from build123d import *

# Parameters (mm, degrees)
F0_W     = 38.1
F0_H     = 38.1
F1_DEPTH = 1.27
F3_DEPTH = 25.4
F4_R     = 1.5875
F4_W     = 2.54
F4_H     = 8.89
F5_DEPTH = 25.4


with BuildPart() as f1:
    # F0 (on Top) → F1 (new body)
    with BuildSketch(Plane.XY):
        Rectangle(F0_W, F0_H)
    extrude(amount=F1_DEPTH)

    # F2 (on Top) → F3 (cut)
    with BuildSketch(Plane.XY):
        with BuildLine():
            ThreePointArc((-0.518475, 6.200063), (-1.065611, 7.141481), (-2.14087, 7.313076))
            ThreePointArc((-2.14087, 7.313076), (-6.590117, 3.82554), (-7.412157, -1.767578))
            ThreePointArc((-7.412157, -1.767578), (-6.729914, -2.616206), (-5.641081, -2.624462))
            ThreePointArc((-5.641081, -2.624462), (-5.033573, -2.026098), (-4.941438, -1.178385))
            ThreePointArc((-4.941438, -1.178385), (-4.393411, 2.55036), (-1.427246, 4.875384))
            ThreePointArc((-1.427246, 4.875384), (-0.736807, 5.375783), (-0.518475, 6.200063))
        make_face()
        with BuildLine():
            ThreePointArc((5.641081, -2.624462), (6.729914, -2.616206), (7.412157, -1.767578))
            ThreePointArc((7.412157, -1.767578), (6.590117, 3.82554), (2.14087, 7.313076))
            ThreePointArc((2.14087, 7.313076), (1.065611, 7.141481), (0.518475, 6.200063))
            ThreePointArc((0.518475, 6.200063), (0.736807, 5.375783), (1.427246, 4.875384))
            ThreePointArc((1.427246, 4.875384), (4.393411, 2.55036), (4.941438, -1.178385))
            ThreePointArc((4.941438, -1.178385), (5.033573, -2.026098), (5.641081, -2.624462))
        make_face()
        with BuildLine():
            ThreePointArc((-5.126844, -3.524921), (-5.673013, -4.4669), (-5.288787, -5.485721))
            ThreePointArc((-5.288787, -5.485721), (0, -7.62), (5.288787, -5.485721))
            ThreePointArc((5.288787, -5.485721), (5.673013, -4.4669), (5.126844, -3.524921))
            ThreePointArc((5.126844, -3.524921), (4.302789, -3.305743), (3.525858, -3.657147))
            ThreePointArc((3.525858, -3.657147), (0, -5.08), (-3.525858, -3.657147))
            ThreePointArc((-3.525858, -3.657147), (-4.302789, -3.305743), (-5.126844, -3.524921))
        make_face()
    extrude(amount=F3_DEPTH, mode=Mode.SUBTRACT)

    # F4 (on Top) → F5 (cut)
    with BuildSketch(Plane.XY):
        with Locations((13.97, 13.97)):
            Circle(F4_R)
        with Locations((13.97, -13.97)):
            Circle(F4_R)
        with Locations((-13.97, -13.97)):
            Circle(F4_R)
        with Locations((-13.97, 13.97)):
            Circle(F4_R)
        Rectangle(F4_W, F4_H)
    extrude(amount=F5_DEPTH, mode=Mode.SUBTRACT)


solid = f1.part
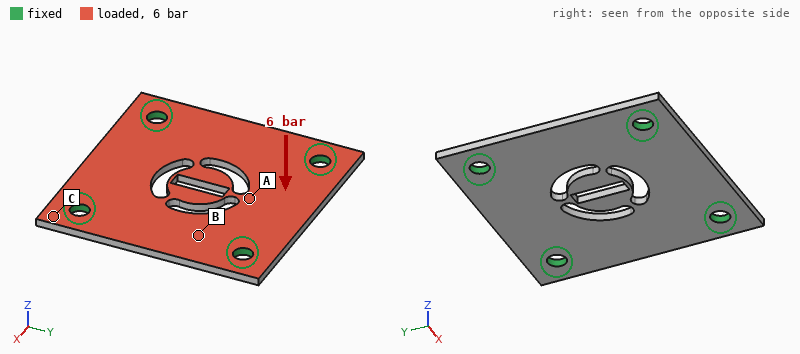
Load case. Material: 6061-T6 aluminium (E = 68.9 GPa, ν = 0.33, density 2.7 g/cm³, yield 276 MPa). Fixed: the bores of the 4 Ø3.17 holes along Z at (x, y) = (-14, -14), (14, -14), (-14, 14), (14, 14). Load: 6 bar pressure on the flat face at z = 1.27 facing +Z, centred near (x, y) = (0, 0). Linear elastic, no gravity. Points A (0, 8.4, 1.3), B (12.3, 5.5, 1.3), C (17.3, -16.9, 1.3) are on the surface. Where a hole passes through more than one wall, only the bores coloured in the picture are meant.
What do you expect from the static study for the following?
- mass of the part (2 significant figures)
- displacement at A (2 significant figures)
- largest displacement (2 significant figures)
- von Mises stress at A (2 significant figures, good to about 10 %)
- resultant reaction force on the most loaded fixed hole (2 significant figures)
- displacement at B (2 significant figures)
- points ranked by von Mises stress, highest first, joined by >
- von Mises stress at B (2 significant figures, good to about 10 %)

4.5 g
0.13 mm
0.18 mm
99 MPa
200 N
0.063 mm
A > B > C
52 MPa
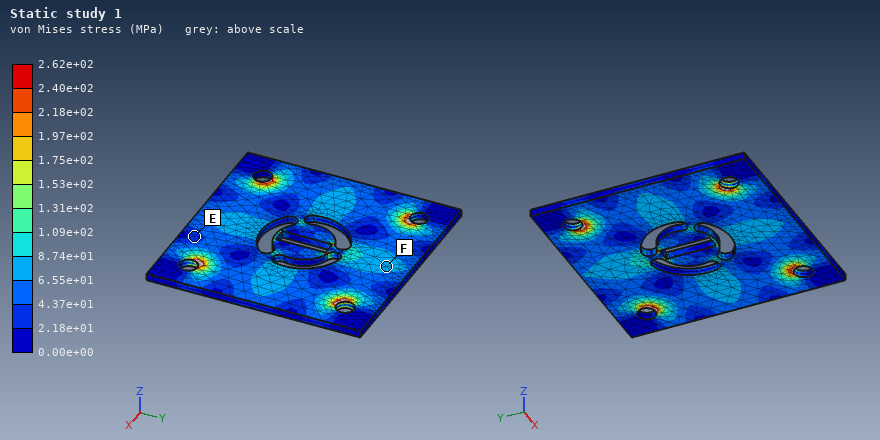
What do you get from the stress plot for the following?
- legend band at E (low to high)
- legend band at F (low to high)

2.18e+01 to 4.37e+01 MPa
6.55e+01 to 8.74e+01 MPa
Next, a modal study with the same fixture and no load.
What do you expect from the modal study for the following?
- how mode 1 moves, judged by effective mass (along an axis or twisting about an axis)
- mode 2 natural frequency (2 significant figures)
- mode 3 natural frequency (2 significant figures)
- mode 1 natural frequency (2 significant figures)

along Z
9900 Hz
9900 Hz
6600 Hz
